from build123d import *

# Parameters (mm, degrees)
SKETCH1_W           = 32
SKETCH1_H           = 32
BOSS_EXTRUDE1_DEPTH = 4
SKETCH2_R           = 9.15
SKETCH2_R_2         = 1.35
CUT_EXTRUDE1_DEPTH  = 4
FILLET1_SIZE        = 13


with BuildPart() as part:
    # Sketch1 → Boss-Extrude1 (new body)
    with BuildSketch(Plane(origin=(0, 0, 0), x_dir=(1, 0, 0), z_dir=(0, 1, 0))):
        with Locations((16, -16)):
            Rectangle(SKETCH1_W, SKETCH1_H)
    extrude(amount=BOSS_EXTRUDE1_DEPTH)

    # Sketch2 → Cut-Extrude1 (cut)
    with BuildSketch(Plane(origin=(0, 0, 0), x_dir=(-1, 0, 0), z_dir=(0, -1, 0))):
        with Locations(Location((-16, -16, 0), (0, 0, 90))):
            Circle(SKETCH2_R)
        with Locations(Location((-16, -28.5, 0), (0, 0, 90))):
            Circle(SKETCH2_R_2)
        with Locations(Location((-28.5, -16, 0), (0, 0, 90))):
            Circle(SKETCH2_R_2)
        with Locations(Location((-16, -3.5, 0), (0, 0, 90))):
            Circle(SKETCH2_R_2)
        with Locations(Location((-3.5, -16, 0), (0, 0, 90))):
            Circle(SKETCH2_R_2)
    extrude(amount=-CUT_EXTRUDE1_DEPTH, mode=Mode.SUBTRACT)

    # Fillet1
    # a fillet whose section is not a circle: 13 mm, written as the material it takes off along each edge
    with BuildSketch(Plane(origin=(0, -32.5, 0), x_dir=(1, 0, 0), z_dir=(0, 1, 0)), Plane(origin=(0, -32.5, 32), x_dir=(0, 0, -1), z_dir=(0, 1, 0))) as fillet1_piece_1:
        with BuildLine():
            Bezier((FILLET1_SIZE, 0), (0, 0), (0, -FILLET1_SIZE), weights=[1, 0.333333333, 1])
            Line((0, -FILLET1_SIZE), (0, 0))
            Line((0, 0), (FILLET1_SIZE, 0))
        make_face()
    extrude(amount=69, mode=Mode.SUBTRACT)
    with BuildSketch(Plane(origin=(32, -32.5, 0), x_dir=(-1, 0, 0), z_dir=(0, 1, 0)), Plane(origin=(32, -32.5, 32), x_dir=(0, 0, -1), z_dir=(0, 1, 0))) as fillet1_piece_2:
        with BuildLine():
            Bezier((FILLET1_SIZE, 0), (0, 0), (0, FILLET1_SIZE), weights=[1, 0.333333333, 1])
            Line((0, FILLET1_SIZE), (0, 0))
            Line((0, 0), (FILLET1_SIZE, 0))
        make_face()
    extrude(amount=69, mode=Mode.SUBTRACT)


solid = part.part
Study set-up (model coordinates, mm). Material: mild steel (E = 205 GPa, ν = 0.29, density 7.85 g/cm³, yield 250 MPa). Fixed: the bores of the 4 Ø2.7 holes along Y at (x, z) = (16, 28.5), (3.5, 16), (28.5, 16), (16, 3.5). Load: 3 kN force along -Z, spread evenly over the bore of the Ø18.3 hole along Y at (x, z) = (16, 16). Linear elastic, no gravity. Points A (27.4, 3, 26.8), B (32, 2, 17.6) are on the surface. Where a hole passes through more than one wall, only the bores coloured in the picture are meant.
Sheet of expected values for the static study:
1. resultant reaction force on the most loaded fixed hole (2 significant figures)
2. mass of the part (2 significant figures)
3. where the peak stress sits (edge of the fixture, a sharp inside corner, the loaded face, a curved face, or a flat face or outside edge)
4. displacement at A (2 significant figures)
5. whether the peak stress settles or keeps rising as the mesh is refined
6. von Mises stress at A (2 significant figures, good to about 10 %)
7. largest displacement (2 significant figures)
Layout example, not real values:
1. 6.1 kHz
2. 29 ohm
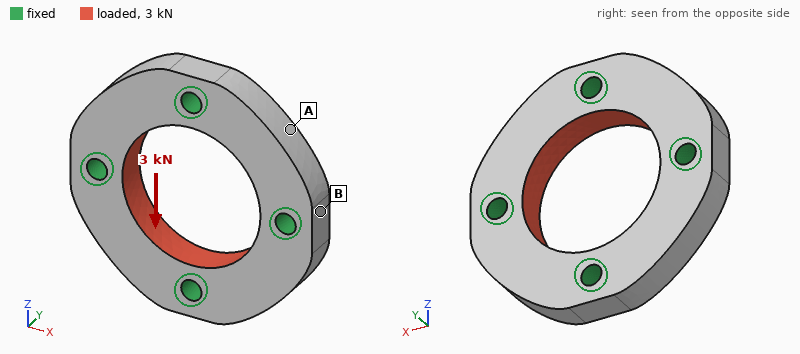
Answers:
1. 860 N
2. 16 g
3. edge of the fixture
4. 0.82 µm
5. keeps rising
6. 17 MPa
7. 1.1 µm
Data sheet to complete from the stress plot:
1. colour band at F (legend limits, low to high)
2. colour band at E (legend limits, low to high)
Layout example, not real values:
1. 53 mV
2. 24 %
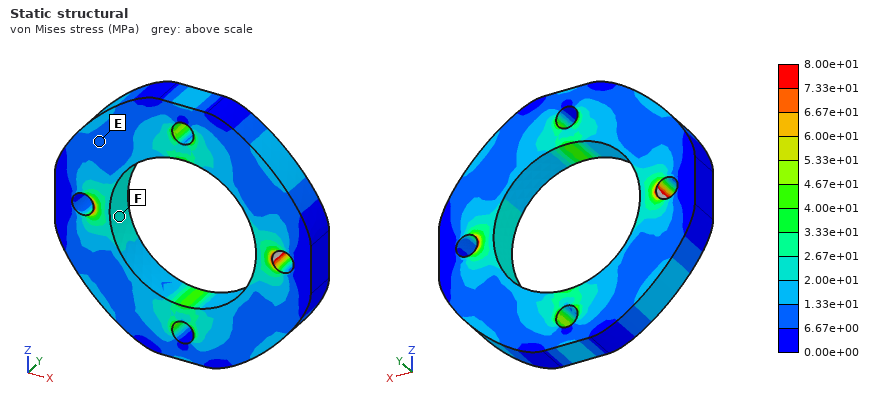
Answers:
1. 2.00e+01 to 2.67e+01 MPa
2. 6.67e+00 to 1.33e+01 MPa
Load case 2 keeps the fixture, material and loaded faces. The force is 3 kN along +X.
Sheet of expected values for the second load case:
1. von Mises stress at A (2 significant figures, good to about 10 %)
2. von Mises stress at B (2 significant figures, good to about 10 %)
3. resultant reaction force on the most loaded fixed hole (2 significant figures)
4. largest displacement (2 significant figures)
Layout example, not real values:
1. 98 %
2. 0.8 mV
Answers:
1. 17 MPa
2. 13 MPa
3. 860 N
4. 1.1 µm
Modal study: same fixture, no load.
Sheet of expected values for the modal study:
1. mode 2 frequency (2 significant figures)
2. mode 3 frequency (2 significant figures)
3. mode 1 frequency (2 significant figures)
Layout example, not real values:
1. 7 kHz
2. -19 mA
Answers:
1. 43 kHz
2. 43 kHz
3. 42 kHz
